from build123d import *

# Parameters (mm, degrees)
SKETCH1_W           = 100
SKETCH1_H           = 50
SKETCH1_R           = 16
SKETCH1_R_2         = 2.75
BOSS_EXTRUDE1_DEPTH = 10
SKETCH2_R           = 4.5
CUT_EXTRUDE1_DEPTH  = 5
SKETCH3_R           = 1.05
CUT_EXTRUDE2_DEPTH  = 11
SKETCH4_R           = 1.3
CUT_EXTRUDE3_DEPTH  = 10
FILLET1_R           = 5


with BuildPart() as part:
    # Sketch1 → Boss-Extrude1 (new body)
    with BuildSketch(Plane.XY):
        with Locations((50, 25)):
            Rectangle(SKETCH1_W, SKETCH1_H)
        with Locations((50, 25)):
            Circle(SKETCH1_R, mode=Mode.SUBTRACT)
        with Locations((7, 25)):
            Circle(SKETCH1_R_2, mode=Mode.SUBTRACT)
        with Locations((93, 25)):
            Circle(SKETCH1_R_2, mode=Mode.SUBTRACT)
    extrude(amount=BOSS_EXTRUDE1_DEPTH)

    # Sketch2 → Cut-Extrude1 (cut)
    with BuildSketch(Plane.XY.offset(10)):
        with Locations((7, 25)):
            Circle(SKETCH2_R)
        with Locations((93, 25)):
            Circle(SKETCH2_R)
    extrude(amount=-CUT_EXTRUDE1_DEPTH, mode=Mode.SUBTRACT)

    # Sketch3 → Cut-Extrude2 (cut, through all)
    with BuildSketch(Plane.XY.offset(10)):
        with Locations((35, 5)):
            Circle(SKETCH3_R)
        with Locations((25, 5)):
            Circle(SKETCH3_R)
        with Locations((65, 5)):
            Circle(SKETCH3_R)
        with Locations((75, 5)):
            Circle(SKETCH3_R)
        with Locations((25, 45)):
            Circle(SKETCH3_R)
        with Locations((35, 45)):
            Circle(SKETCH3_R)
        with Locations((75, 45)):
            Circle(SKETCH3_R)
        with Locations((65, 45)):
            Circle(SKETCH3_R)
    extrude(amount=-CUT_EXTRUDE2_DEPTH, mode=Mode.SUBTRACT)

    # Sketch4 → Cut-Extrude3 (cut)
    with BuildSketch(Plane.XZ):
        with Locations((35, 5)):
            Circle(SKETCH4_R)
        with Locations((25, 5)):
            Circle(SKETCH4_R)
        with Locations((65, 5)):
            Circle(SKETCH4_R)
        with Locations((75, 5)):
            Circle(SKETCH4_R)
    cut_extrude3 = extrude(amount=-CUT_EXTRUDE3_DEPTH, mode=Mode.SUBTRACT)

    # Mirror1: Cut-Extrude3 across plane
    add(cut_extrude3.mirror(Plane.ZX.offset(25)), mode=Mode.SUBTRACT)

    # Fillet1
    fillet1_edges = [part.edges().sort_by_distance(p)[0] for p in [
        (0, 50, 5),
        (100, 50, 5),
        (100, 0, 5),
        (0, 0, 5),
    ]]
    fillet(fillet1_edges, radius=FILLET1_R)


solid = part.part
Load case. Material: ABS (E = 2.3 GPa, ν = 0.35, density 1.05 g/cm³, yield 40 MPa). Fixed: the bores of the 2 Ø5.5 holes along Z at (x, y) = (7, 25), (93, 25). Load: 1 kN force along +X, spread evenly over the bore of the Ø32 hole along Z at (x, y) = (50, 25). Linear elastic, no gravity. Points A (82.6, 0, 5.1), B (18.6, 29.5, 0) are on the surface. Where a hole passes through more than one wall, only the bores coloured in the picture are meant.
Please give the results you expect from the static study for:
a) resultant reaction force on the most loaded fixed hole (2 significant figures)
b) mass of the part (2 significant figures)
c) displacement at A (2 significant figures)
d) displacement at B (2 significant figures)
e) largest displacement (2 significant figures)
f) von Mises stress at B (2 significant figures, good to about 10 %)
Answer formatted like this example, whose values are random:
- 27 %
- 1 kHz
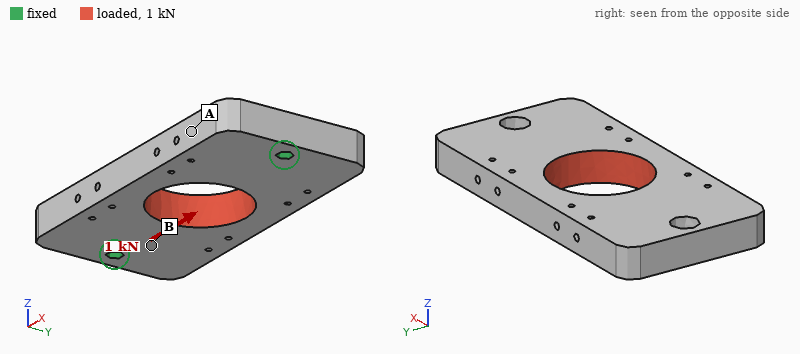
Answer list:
- 500 N
- 42 g
- 38 µm
- 21 µm
- 51 µm
- 3.0 MPa
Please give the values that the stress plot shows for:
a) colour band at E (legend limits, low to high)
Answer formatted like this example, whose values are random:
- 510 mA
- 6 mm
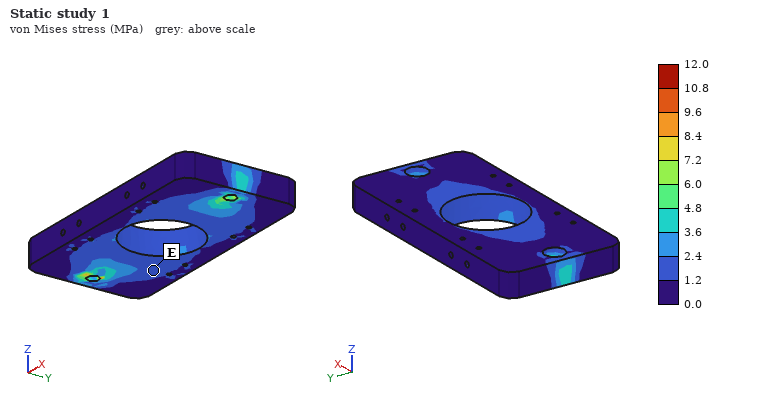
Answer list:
- 1.2 to 2.4 MPa
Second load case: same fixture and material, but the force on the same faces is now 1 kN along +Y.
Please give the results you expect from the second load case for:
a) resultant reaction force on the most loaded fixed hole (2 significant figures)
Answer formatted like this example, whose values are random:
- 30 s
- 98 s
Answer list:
- 500 N
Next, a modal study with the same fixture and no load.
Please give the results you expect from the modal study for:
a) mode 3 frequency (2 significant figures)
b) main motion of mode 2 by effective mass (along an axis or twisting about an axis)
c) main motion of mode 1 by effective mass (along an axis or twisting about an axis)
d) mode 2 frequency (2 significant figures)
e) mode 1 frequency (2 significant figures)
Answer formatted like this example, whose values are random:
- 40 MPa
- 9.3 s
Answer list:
- 2000 Hz
- along Z
- twisting about X
- 1200 Hz
- 1000 Hz
